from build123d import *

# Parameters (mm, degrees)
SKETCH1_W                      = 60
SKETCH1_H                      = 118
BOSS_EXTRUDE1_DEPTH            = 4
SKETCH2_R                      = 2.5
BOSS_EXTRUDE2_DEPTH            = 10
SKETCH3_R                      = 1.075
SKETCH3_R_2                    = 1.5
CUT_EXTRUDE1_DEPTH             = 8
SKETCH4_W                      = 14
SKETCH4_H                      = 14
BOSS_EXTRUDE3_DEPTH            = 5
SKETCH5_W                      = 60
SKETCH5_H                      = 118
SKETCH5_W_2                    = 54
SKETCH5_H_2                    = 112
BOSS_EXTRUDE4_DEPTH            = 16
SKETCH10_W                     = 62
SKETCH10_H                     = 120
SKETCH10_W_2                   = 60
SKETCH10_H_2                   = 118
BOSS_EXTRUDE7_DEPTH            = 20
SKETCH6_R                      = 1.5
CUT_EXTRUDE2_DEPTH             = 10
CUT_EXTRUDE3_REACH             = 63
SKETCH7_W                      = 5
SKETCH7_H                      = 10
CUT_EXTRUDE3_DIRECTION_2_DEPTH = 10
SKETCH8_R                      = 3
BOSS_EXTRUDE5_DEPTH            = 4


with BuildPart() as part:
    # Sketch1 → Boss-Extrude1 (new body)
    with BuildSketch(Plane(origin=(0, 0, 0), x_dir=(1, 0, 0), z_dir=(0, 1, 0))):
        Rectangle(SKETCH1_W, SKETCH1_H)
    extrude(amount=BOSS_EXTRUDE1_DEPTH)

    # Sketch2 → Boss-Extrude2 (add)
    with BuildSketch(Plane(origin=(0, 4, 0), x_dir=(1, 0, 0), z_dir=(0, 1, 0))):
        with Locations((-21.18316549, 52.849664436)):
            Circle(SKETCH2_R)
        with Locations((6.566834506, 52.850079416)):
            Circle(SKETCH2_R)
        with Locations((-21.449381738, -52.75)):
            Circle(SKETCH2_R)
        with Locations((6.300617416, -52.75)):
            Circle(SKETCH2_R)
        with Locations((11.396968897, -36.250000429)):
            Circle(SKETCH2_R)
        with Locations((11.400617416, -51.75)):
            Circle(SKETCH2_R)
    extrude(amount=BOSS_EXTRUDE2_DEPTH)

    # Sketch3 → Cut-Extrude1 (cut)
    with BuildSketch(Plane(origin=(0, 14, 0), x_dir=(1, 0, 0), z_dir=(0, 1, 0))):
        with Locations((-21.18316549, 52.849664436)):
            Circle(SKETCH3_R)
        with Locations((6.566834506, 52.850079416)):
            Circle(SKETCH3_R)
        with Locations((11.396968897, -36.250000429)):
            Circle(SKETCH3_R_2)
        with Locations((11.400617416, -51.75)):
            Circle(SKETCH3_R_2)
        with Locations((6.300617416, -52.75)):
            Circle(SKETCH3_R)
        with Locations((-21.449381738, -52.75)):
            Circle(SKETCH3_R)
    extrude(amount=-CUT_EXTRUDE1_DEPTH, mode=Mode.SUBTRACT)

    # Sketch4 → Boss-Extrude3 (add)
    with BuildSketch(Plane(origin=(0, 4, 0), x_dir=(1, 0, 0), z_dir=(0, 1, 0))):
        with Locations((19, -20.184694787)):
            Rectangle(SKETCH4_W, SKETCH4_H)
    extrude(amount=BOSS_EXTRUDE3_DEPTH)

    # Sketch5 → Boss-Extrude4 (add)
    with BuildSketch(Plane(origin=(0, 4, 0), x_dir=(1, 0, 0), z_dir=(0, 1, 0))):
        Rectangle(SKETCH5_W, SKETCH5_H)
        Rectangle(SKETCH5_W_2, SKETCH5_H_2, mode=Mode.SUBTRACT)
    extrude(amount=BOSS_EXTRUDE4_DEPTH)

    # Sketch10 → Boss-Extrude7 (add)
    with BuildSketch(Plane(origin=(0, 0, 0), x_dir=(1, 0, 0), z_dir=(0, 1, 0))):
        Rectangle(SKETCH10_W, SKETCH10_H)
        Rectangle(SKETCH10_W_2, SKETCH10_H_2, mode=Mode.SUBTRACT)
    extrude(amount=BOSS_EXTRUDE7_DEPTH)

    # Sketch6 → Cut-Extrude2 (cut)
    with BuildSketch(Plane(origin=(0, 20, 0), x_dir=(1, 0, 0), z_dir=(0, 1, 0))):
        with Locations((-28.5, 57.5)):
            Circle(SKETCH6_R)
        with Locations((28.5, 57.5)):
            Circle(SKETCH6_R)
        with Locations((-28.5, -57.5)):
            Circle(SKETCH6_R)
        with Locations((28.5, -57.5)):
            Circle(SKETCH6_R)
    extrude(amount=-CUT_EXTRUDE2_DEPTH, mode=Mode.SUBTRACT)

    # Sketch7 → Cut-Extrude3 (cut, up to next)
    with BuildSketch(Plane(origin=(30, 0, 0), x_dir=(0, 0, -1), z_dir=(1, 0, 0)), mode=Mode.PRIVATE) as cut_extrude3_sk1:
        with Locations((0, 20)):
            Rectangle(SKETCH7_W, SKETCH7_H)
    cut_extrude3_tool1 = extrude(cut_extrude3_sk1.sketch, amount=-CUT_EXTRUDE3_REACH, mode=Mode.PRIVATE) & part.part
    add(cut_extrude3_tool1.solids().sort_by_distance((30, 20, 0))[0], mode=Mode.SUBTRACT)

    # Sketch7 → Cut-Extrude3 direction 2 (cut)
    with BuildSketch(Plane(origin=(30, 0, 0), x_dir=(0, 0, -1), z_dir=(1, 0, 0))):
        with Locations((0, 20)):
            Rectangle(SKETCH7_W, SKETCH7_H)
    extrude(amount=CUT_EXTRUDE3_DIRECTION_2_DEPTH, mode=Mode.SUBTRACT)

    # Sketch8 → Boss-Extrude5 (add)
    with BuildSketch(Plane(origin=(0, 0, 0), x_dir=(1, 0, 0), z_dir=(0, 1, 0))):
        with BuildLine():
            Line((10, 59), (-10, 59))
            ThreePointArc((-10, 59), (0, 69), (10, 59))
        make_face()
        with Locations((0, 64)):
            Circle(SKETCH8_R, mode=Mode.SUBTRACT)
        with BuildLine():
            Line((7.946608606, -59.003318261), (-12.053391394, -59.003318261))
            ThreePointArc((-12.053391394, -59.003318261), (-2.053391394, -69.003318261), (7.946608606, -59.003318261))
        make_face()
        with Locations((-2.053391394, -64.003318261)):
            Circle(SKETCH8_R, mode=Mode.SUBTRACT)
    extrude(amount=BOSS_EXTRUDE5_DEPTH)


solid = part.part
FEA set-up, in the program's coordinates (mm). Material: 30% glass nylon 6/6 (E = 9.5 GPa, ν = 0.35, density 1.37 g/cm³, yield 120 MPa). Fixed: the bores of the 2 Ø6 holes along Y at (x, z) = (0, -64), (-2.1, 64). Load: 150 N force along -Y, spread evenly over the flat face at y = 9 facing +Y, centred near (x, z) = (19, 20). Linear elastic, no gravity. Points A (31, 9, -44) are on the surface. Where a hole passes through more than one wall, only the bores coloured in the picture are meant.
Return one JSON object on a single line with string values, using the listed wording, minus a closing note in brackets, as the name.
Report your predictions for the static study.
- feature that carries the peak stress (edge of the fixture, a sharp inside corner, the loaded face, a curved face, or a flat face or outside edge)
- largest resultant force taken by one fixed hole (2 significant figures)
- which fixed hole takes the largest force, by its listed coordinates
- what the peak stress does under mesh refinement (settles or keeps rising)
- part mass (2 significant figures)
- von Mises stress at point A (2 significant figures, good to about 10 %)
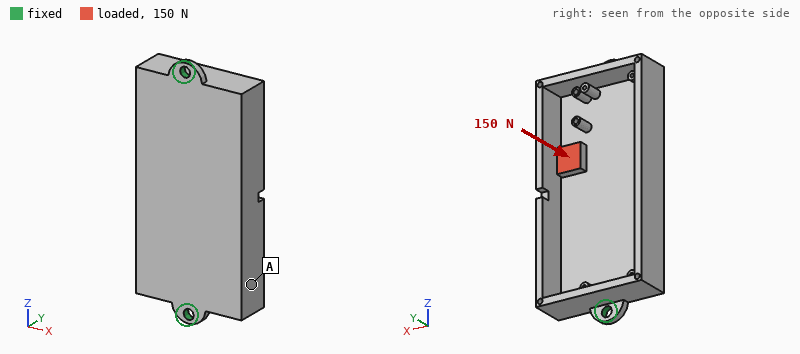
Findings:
{"feature that carries the peak stress": "edge of the fixture", "largest resultant force taken by one fixed hole": "110 N", "which fixed hole takes the largest force, by its listed coordinates": "(-2.1, 64)", "what the peak stress does under mesh refinement": "keeps rising", "part mass": "75 g", "von Mises stress at point A": "1.7 MPa"}
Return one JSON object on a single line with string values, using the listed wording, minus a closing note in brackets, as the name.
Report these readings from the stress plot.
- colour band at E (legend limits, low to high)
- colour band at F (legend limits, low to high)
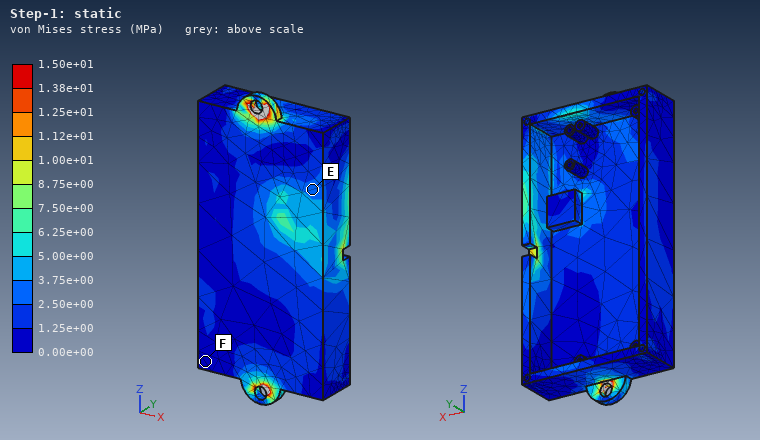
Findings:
{"colour band at E": "2.50e+00 to 3.75e+00 MPa", "colour band at F": "0.00e+00 to 1.25e+00 MPa"}
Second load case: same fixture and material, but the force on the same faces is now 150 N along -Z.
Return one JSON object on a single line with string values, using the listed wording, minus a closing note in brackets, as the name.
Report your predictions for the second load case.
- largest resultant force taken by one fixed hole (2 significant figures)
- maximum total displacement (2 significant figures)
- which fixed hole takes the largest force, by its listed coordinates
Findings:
{"largest resultant force taken by one fixed hole": "84 N", "maximum total displacement": "17 µm", "which fixed hole takes the largest force, by its listed coordinates": "(-2.1, 64)"}
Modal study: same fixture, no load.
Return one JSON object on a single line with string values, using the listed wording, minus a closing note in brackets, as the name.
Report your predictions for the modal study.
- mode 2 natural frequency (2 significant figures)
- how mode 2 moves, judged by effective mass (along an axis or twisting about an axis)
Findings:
{"mode 2 natural frequency": "1200 Hz", "how mode 2 moves, judged by effective mass": "along Y"}
